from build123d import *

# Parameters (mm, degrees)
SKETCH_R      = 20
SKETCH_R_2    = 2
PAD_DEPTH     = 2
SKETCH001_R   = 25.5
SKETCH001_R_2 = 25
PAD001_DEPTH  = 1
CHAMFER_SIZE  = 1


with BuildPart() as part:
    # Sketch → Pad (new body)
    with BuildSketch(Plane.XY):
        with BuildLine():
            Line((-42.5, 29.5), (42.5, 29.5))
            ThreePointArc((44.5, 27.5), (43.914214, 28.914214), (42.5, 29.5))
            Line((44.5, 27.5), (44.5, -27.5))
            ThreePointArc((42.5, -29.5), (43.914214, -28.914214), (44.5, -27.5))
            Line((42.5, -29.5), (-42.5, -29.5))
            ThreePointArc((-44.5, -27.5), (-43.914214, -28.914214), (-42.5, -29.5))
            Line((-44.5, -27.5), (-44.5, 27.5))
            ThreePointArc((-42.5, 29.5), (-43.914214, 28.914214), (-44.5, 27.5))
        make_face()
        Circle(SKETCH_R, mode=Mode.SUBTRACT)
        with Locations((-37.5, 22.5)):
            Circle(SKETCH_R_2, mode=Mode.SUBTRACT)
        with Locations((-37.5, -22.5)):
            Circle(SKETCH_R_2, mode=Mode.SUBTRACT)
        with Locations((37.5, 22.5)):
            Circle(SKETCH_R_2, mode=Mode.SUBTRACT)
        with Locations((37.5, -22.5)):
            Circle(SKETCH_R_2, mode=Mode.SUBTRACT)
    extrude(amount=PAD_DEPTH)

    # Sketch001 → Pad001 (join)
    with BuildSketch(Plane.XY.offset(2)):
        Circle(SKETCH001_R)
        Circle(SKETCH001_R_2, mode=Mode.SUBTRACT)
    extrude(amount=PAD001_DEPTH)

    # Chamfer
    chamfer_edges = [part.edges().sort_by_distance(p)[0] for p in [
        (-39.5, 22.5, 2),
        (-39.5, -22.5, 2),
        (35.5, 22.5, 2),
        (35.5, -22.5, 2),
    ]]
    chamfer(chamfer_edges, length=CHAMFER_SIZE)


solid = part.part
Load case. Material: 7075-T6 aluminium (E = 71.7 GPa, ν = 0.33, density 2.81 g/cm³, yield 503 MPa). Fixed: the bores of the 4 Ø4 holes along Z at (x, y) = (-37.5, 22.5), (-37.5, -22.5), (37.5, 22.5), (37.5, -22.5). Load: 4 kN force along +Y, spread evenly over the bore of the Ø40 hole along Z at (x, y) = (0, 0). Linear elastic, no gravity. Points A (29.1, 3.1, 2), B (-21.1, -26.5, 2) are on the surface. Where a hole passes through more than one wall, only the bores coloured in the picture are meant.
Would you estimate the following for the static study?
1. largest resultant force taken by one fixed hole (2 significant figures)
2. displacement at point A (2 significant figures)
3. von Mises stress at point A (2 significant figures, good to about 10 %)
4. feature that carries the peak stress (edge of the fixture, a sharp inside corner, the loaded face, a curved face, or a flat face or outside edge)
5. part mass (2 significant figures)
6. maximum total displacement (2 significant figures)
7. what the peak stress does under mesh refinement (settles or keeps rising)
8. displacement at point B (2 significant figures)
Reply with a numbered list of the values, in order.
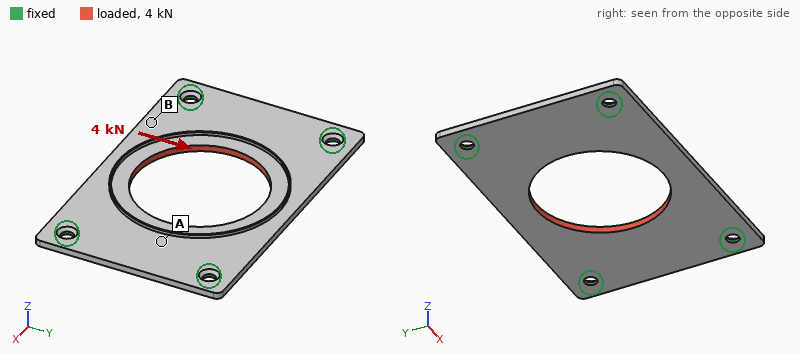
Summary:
1. 1.1 kN
2. 12 µm
3. 47 MPa
4. edge of the fixture
5. 22 g
6. 44 µm
7. keeps rising
8. 20 µm
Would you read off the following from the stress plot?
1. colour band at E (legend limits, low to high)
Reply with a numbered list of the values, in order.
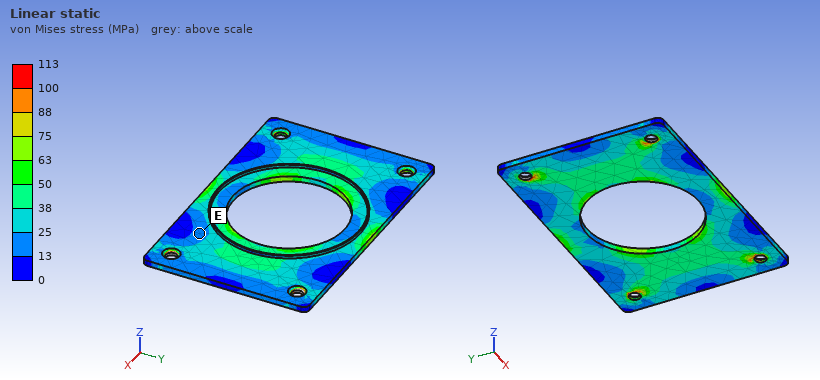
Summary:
1. 13 to 25 MPa
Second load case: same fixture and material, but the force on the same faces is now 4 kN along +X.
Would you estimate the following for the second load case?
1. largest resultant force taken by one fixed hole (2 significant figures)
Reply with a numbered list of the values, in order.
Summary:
1. 1.0 kN
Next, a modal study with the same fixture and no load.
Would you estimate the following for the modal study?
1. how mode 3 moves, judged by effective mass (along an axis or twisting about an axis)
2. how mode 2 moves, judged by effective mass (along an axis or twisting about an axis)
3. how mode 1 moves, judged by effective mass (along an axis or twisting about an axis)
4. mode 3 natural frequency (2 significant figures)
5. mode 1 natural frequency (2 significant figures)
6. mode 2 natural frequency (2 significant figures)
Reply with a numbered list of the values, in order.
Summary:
1. twisting about Y
2. twisting about X
3. along Z
4. 3700 Hz
5. 1900 Hz
6. 2300 Hz
